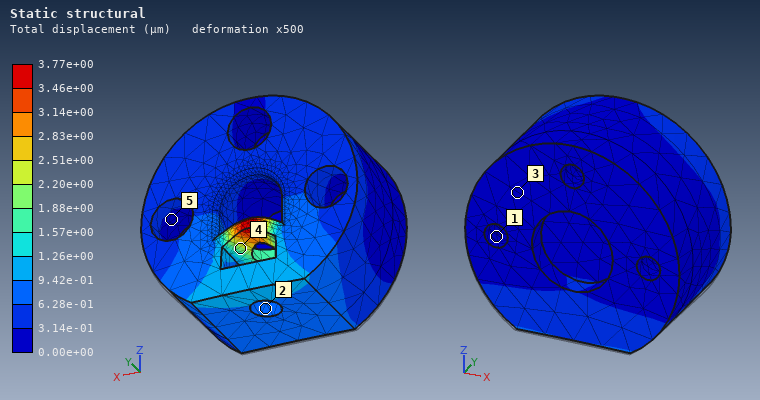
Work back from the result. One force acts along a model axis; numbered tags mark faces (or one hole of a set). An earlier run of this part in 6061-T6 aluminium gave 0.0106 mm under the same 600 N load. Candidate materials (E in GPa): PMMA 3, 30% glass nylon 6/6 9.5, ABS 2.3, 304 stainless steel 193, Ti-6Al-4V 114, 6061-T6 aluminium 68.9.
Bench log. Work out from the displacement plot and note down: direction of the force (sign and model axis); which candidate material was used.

+Z
304 stainless steel
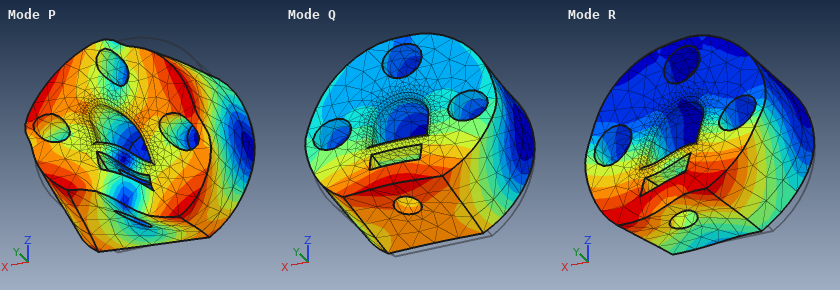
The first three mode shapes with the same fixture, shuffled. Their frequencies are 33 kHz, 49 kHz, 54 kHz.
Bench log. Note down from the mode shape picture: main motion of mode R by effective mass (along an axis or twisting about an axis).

along X
